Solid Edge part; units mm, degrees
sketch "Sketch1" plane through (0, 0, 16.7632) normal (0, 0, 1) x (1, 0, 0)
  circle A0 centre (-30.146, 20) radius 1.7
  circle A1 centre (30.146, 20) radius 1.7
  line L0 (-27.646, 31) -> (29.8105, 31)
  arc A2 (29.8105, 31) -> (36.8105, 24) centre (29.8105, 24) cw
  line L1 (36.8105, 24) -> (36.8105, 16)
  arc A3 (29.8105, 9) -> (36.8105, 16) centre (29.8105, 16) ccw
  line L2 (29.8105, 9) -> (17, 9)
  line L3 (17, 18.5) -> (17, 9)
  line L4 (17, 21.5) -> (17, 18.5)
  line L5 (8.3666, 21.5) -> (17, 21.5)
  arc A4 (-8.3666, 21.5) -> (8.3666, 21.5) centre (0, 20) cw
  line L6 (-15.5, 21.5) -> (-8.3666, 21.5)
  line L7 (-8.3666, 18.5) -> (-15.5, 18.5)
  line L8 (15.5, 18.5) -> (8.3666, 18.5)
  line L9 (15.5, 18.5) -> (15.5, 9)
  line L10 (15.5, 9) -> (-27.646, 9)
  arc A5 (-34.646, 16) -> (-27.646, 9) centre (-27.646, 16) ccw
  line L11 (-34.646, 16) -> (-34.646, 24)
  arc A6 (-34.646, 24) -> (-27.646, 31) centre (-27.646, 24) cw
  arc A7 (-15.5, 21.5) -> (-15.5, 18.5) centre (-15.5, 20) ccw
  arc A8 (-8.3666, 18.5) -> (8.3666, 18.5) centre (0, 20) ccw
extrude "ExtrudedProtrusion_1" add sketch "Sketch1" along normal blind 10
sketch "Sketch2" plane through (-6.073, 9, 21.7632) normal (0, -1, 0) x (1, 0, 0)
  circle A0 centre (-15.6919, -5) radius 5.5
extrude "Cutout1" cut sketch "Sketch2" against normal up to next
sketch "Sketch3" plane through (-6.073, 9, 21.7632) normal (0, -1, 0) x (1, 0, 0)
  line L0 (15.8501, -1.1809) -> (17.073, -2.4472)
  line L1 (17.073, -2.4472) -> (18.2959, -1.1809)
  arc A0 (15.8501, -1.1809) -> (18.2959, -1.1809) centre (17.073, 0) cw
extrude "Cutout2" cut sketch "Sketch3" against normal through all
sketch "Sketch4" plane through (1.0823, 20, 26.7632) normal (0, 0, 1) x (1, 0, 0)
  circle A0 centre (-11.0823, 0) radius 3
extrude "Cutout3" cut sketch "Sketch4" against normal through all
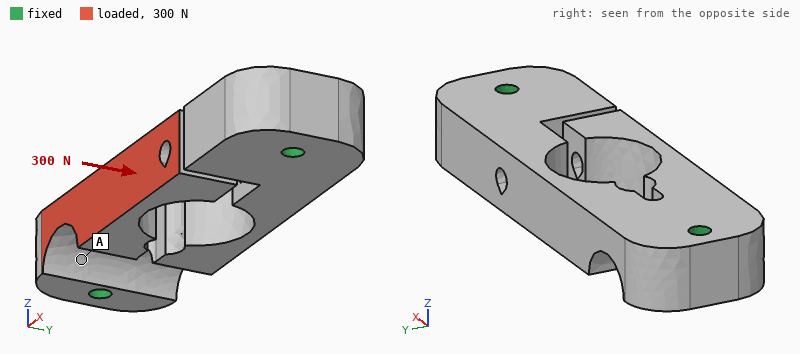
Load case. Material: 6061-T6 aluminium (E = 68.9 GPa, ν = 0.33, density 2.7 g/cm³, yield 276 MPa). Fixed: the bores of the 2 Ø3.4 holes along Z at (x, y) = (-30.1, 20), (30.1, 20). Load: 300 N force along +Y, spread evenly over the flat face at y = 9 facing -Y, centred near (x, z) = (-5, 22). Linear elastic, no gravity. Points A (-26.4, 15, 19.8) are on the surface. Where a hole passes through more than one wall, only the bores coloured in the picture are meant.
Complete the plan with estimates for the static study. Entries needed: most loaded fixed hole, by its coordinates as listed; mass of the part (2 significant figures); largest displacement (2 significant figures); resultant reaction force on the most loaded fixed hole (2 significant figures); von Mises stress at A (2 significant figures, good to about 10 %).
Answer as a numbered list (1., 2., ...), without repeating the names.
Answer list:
1. (-30.1, 20)
2. 29 g
3. 0.23 mm
4. 300 N
5. 10 MPa
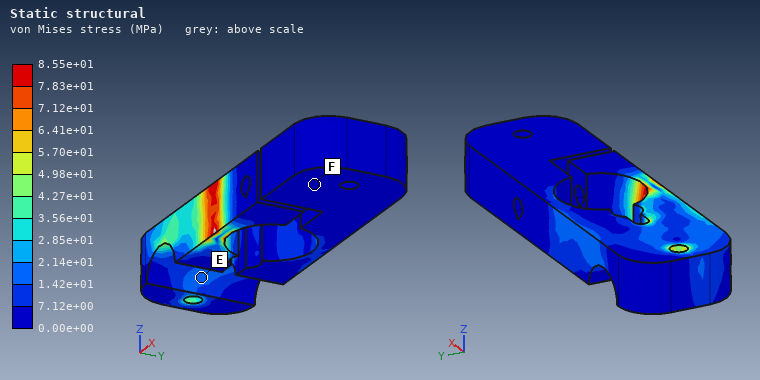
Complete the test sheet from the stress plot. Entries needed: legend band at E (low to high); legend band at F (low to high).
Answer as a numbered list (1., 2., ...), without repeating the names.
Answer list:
1. 1.42e+01 to 2.14e+01 MPa
2. 0.00e+00 to 7.12e+00 MPa
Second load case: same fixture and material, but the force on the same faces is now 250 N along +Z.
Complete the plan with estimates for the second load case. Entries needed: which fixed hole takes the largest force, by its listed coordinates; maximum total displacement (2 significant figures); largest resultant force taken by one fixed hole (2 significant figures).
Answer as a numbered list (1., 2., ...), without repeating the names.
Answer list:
1. (-30.1, 20)
2. 0.23 mm
3. 220 N
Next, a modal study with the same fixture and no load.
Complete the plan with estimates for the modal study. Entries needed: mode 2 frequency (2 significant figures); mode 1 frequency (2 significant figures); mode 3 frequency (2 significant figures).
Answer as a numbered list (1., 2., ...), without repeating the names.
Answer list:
1. 2600 Hz
2. 2500 Hz
3. 8500 Hz
